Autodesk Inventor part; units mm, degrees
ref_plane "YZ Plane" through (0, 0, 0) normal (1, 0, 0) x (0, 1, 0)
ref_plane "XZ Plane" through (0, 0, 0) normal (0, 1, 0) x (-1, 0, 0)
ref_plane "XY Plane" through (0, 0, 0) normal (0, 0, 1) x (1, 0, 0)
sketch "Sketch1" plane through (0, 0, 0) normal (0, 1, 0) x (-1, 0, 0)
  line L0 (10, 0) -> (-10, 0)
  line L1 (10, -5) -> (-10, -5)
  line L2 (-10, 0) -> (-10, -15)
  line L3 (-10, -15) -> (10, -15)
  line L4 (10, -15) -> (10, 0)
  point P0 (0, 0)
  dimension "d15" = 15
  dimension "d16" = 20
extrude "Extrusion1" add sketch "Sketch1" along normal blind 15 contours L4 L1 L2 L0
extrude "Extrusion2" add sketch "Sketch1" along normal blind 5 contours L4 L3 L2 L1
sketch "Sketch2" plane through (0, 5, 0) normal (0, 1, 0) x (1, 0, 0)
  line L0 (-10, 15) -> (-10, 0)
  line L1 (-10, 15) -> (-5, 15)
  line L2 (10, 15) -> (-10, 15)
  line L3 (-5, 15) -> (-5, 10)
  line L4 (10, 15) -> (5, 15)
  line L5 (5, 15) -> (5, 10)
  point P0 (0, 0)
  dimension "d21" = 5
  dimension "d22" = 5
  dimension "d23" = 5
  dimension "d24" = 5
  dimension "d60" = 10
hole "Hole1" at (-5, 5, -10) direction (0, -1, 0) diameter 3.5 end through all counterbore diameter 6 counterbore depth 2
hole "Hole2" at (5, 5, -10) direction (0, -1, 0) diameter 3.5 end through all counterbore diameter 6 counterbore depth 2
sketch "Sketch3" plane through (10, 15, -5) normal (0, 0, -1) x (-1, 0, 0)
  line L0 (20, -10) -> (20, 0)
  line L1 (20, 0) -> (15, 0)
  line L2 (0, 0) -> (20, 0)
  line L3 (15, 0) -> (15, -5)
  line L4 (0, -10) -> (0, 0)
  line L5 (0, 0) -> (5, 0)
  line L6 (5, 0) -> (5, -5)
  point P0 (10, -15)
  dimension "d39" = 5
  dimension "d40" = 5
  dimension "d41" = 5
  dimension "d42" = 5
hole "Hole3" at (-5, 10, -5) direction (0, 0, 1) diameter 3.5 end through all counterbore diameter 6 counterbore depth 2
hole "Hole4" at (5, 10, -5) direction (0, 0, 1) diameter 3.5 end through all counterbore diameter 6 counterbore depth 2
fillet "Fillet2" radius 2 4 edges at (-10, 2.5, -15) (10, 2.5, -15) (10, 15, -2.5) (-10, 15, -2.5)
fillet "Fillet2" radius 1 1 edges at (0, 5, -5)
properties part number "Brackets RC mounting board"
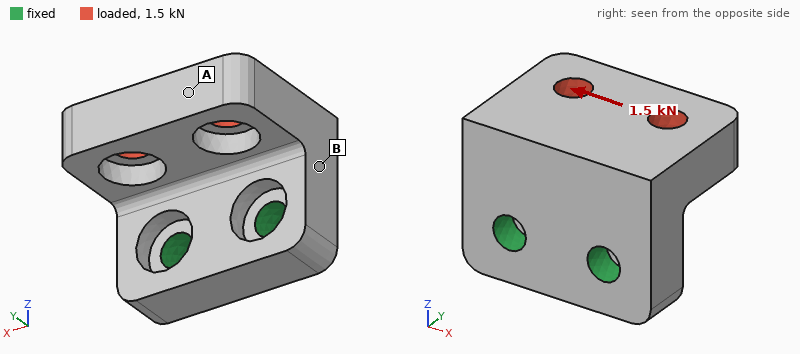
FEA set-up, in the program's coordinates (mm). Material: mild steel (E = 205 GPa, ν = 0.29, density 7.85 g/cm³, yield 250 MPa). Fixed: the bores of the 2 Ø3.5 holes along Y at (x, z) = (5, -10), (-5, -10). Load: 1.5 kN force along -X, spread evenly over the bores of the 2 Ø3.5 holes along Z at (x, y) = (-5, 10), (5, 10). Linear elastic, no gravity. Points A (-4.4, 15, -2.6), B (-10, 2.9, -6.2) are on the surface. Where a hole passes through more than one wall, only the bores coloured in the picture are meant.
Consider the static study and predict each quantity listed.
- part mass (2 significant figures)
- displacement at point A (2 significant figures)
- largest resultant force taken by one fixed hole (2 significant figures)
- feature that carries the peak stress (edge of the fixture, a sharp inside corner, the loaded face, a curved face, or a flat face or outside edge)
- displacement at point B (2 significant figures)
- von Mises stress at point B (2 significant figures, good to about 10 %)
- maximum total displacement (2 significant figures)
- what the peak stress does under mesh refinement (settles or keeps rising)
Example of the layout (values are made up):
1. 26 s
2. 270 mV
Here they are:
1. 17 g
2. 14 µm
3. 1.6 kN
4. edge of the fixture
5. 5.1 µm
6. 63 MPa
7. 15 µm
8. keeps rising
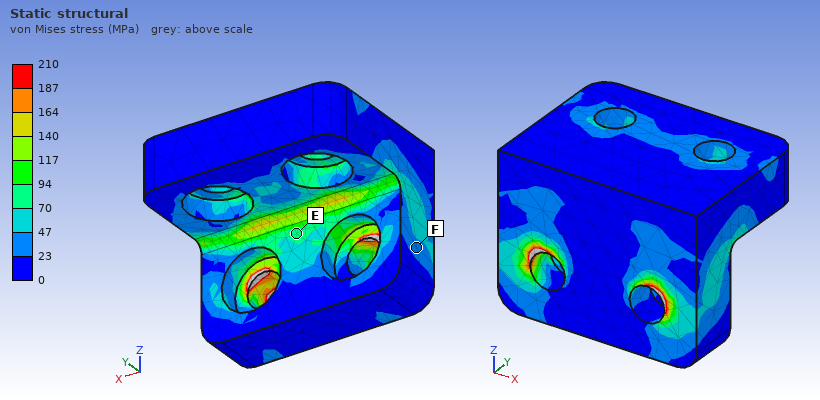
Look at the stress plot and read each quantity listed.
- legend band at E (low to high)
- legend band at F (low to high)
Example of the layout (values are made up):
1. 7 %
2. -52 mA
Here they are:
1. 70 to 94 MPa
2. 23 to 47 MPa
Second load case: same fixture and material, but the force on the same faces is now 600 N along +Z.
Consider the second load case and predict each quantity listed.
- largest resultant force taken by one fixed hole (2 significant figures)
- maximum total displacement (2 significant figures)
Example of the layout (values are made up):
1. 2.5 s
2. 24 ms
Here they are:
1. 300 N
2. 21 µm
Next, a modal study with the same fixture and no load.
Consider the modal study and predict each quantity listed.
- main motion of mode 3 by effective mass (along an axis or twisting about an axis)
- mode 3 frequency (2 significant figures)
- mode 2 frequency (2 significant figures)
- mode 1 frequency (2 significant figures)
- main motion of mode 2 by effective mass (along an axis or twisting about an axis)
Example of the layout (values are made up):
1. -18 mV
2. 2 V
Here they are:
1. along X
2. 31 kHz
3. 19 kHz
4. 11 kHz
5. along X
